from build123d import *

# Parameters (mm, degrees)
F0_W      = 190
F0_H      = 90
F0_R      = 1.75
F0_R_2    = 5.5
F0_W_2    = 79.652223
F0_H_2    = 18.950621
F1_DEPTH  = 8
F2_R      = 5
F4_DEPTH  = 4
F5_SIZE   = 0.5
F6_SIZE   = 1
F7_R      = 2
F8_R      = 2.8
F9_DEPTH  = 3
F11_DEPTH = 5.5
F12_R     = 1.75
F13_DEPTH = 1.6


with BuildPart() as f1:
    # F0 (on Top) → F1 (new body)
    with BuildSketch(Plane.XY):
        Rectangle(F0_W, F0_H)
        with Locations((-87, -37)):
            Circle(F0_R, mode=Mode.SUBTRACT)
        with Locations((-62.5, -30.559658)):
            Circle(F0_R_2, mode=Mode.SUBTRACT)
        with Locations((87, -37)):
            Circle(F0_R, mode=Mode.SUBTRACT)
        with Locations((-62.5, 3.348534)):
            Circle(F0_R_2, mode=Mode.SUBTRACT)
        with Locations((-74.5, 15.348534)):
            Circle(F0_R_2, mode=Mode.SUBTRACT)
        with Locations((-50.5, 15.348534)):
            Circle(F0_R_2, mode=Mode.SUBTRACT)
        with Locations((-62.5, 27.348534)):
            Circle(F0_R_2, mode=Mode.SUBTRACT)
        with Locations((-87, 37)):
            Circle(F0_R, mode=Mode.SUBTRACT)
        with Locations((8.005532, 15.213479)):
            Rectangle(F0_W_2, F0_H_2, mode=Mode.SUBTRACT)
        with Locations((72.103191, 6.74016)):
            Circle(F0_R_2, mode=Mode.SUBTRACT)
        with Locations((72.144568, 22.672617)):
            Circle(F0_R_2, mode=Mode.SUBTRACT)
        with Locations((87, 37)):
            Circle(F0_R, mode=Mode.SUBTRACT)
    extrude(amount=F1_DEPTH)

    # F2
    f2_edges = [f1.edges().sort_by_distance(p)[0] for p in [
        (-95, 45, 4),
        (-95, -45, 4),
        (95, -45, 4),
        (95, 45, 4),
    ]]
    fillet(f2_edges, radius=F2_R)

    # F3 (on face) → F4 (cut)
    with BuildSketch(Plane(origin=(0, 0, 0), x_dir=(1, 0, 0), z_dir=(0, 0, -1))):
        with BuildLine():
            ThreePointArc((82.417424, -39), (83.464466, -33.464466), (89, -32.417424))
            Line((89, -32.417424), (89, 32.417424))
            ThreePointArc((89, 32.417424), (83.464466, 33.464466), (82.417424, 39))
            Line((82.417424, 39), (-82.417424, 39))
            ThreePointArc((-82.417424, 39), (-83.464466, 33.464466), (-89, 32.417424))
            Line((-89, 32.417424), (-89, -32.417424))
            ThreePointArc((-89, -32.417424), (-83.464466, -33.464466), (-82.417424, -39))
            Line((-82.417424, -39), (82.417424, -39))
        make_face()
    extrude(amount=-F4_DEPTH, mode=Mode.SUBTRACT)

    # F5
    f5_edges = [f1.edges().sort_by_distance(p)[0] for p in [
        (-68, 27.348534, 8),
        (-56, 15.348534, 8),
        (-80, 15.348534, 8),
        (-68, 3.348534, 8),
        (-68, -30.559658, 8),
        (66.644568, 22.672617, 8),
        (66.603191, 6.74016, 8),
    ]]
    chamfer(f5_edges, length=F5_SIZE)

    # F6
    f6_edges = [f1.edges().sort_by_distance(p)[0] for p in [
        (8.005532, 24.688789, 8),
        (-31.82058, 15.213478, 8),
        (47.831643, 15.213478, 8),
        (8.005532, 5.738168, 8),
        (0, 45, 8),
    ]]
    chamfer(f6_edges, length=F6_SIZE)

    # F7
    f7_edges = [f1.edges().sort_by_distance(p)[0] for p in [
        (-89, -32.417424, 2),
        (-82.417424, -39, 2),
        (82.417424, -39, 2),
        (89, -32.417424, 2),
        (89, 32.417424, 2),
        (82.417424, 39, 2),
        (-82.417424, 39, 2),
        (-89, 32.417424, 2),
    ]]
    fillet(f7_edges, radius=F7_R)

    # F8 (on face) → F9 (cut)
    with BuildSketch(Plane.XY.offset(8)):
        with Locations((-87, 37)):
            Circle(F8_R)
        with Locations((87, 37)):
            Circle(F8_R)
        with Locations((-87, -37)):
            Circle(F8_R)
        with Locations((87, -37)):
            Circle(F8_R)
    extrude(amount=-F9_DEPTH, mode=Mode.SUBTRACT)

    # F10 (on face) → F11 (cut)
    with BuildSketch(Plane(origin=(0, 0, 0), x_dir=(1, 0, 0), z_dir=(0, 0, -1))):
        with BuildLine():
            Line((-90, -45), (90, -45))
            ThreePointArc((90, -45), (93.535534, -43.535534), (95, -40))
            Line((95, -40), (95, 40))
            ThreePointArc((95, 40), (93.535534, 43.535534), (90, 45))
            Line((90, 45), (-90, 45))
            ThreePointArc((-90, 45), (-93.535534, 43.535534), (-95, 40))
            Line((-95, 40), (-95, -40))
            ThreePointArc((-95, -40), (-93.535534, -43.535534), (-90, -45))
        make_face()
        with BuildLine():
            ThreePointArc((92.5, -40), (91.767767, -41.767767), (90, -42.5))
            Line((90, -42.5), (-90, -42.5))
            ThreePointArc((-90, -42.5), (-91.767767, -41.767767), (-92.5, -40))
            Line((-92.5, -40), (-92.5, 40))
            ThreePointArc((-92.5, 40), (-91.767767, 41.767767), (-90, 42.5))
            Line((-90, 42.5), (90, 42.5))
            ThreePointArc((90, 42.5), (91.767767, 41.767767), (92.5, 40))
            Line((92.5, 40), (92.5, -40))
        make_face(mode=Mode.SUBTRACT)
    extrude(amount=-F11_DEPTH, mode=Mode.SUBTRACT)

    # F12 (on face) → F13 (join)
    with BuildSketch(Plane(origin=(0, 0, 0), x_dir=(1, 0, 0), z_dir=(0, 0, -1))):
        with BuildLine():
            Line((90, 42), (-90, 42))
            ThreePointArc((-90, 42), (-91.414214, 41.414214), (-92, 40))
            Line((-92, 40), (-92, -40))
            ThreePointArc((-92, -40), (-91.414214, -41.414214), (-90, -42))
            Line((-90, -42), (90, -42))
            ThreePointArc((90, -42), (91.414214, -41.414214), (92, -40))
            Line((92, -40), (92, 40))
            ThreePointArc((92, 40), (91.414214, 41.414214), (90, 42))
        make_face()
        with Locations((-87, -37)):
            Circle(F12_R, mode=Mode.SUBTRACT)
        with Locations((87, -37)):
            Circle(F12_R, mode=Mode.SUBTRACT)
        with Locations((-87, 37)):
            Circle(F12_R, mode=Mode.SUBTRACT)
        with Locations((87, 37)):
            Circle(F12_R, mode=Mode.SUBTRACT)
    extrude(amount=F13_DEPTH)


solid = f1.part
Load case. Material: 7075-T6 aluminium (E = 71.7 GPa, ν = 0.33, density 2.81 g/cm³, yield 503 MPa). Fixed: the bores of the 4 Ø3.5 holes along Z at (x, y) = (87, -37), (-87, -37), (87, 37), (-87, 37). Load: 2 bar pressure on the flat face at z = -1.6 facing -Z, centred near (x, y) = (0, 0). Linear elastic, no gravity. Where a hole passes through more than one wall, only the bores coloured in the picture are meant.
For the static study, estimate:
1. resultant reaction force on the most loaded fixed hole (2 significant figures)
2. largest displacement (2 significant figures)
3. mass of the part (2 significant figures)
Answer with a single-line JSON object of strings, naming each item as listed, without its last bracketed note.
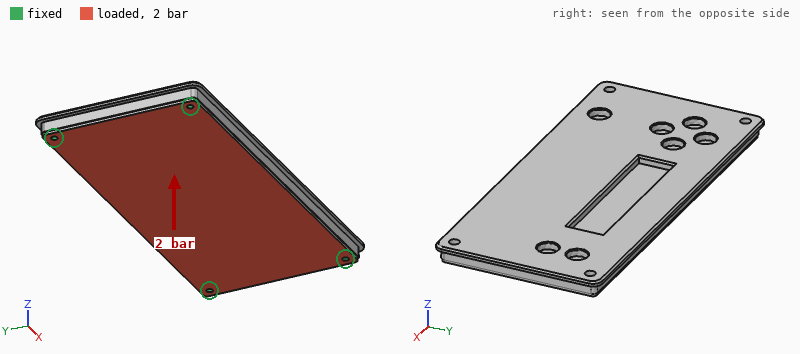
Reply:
{"resultant reaction force on the most loaded fixed hole": "960 N", "largest displacement": "1.1 mm", "mass of the part": "250 g"}
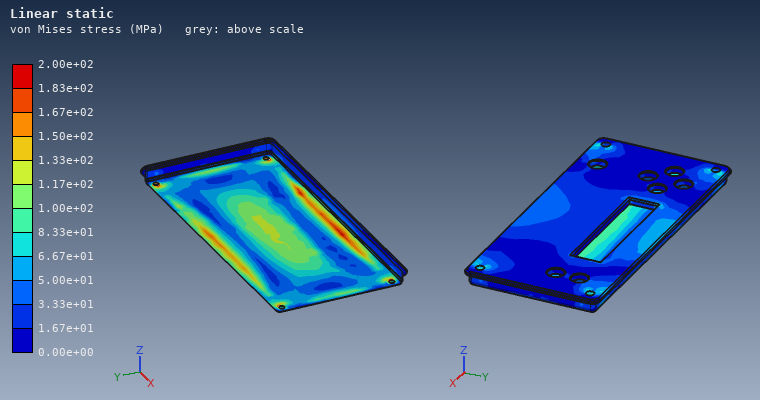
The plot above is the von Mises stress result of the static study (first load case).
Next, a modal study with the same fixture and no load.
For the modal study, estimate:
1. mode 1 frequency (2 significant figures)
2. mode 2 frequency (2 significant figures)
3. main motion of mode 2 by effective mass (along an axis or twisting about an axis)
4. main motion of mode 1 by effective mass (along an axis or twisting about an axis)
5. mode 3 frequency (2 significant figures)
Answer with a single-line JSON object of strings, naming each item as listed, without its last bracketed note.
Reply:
{"mode 1 frequency": "1000 Hz", "mode 2 frequency": "1600 Hz", "main motion of mode 2 by effective mass": "twisting about X", "main motion of mode 1 by effective mass": "along Z", "mode 3 frequency": "1800 Hz"}
